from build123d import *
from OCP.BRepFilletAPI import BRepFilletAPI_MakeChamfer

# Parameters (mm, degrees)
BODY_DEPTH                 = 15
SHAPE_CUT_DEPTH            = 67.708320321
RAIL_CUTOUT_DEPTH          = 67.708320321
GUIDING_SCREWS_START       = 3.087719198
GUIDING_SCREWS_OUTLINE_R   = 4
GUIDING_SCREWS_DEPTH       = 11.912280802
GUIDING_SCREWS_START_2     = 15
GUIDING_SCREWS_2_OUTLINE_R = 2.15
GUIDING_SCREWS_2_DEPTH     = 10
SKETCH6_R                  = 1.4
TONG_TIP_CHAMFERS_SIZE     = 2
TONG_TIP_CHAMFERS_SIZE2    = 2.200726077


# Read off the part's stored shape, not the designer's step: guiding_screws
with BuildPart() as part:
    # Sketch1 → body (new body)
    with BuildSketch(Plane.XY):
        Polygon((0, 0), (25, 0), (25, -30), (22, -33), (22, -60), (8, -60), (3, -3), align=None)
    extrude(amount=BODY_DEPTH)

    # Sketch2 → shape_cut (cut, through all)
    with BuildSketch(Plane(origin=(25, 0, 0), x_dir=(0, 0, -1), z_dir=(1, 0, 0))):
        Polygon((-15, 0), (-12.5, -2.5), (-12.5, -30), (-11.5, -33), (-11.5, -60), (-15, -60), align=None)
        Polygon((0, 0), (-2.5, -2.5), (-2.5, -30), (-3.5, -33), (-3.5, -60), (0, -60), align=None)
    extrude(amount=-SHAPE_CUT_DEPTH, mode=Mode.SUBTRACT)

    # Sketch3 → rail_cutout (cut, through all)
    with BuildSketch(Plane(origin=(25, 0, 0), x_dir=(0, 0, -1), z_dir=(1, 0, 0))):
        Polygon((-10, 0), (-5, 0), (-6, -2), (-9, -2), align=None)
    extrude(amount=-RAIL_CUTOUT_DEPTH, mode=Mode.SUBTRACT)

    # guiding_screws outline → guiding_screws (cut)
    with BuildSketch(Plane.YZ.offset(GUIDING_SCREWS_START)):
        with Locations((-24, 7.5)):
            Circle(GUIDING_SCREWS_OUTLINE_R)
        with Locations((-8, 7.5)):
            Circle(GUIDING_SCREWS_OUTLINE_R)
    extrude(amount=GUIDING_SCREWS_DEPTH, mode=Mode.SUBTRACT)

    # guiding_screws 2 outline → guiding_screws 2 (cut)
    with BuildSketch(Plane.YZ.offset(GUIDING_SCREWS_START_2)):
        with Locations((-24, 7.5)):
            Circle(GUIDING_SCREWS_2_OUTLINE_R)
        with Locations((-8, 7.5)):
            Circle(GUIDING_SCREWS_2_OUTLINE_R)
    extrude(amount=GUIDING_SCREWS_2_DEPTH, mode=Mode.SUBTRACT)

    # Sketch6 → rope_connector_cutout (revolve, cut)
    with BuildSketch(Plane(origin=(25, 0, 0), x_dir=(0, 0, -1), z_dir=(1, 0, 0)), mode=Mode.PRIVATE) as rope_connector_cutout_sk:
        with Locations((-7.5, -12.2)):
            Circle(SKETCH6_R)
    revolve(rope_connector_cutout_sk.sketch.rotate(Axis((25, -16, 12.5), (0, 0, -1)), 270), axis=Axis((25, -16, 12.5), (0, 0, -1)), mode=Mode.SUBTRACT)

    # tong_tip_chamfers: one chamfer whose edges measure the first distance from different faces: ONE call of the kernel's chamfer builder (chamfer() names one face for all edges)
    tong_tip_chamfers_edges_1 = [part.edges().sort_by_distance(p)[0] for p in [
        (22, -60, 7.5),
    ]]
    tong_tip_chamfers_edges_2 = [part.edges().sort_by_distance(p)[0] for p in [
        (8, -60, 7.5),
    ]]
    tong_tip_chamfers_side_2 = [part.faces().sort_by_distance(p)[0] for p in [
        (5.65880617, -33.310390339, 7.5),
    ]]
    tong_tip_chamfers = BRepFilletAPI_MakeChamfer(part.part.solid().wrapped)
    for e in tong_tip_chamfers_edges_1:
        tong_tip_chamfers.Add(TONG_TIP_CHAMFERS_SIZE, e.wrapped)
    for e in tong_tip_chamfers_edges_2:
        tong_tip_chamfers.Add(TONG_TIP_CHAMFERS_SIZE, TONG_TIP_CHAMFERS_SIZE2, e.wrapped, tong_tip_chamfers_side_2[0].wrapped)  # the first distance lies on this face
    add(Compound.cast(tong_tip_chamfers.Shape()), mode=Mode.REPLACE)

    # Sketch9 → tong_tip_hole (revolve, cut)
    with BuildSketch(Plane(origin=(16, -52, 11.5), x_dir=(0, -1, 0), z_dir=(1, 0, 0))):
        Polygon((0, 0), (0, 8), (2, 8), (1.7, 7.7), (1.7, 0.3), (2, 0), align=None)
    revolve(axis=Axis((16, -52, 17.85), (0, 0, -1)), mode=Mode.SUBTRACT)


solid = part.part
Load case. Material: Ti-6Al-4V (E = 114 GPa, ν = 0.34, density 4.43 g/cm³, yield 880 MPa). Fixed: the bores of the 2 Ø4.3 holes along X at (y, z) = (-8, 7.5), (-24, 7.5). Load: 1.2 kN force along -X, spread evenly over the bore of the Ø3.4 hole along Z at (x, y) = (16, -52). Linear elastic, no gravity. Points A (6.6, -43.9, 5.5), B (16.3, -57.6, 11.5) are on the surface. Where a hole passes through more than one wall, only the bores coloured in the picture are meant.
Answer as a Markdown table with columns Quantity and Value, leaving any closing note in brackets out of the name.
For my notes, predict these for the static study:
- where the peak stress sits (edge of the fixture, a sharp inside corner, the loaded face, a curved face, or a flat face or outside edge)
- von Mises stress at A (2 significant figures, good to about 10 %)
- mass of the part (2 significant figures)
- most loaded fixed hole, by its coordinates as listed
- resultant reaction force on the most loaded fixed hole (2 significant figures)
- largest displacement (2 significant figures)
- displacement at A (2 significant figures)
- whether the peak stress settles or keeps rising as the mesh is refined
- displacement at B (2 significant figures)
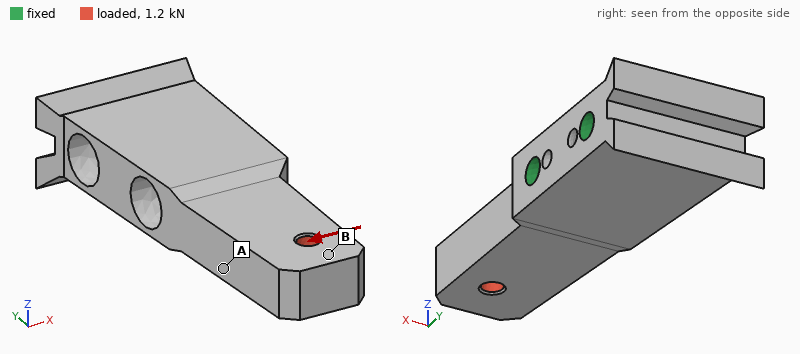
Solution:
| Quantity | Value |
|---|---|
| where the peak stress sits | a sharp inside corner |
| von Mises stress at A | 34 MPa |
| mass of the part | 38 g |
| most loaded fixed hole, by its coordinates as listed | (-24, 7.5) |
| resultant reaction force on the most loaded fixed hole | 2.2 kN |
| largest displacement | 61 µm |
| displacement at A | 32 µm |
| whether the peak stress settles or keeps rising as the mesh is refined | keeps rising |
| displacement at B | 55 µm |
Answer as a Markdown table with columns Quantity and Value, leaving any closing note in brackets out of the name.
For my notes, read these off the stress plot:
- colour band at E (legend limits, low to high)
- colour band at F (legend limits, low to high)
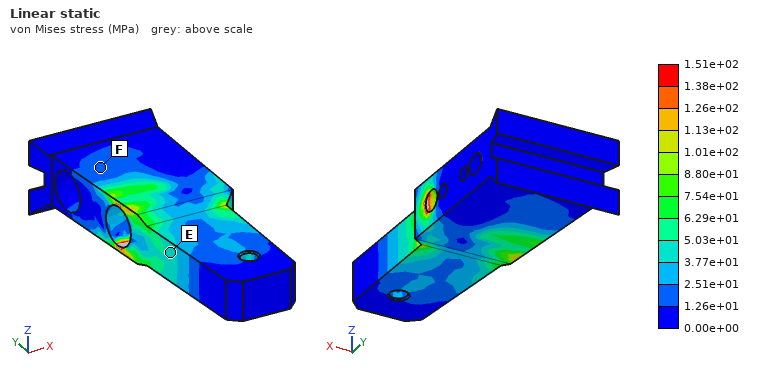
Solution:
| Quantity | Value |
|---|---|
| colour band at E | 3.77e+01 to 5.03e+01 MPa |
| colour band at F | 1.26e+01 to 2.51e+01 MPa |
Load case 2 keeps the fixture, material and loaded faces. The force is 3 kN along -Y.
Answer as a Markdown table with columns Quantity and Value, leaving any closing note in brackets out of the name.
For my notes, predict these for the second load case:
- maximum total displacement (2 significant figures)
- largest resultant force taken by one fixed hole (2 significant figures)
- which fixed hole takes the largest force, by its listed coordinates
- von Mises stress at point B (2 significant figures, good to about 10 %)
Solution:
| Quantity | Value |
|---|---|
| maximum total displacement | 9.4 µm |
| largest resultant force taken by one fixed hole | 2.6 kN |
| which fixed hole takes the largest force, by its listed coordinates | (-24, 7.5) |
| von Mises stress at point B | 12 MPa |
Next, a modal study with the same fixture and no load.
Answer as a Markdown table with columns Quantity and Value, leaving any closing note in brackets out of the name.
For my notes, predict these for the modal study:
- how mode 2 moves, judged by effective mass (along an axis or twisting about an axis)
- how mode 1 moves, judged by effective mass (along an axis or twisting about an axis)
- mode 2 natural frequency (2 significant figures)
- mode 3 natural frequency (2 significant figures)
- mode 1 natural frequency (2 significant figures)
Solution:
| Quantity | Value |
|---|---|
| how mode 2 moves, judged by effective mass | along X |
| how mode 1 moves, judged by effective mass | along Z |
| mode 2 natural frequency | 8400 Hz |
| mode 3 natural frequency | 17 kHz |
| mode 1 natural frequency | 5600 Hz |
